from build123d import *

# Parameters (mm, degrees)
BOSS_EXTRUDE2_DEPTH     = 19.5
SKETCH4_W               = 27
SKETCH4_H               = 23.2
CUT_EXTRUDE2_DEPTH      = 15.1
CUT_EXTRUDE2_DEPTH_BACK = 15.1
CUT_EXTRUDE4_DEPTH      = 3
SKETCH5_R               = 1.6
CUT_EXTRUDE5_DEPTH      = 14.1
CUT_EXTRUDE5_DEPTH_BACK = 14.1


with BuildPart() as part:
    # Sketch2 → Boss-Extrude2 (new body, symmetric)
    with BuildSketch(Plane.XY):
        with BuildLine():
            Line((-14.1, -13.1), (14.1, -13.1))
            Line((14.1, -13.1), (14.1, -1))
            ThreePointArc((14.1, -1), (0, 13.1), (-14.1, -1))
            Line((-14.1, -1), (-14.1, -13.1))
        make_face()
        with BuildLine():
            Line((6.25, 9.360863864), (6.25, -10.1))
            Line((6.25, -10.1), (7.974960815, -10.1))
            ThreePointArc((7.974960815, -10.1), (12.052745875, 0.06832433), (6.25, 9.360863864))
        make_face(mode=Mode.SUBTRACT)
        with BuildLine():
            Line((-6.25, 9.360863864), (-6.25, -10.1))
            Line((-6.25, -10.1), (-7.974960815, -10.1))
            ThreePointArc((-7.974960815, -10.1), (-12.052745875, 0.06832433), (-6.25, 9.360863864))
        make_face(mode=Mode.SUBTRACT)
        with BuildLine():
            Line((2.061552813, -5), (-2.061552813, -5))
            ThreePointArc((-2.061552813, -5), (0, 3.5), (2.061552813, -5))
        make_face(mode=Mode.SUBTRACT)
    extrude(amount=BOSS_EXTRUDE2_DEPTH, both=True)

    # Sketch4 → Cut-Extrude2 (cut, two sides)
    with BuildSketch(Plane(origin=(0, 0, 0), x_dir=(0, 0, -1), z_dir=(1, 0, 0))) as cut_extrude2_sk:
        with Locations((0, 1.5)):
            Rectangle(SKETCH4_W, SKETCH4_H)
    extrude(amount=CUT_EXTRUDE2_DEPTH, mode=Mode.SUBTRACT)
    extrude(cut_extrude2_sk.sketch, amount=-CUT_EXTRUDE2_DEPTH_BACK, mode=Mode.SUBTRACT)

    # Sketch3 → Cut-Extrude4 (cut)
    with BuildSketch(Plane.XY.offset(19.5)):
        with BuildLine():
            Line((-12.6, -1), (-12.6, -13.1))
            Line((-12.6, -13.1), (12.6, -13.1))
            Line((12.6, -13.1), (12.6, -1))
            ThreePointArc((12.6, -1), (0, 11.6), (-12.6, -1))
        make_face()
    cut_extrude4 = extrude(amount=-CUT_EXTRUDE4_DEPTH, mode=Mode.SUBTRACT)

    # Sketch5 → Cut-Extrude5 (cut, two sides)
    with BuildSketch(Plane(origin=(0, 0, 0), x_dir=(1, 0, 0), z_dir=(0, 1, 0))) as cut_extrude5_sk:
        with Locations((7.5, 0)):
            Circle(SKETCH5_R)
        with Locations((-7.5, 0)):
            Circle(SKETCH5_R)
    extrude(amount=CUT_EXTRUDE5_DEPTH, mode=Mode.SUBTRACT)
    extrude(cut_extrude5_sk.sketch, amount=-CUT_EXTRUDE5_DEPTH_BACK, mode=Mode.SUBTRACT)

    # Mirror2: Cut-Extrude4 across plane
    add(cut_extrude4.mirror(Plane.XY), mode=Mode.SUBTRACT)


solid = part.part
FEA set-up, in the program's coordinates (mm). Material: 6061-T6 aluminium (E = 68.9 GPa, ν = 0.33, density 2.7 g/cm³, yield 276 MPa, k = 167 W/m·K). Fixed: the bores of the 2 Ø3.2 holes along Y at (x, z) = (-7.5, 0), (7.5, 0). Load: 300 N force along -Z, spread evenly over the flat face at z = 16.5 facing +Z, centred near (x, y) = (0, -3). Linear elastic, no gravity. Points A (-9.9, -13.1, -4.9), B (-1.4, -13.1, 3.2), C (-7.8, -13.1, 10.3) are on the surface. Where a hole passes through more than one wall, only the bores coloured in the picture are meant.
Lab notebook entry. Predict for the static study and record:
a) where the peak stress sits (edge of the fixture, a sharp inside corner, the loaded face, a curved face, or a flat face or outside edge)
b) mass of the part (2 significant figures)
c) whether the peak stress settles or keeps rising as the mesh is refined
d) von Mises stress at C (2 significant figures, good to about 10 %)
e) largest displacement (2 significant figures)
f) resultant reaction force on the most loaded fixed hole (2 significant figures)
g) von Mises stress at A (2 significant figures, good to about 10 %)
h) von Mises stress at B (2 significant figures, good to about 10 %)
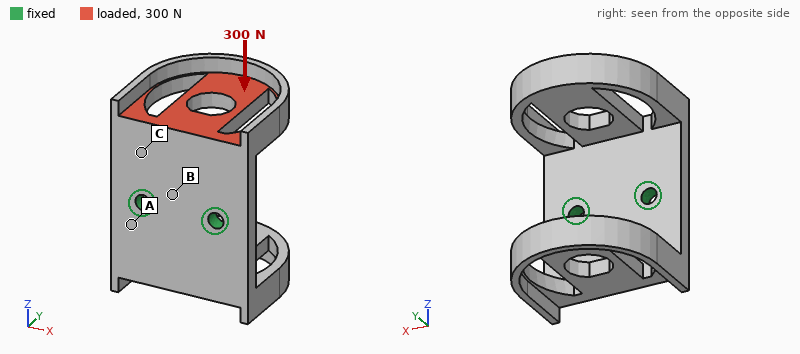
edge of the fixture
14 g
keeps rising
52 MPa
0.32 mm
150 N
7.1 MPa
44 MPa
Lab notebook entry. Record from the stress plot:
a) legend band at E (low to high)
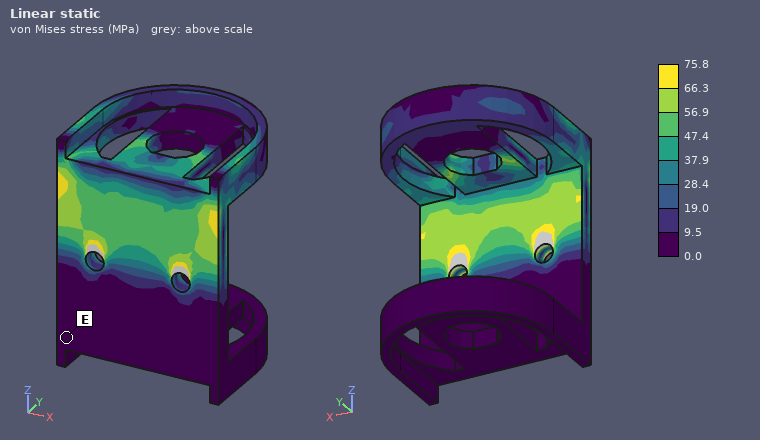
0.0 to 9.5 MPa
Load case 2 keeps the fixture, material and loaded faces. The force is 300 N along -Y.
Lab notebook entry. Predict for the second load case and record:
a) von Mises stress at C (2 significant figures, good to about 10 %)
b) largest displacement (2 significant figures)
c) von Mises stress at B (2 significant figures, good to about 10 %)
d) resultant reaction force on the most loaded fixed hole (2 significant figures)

39 MPa
0.26 mm
65 MPa
150 N
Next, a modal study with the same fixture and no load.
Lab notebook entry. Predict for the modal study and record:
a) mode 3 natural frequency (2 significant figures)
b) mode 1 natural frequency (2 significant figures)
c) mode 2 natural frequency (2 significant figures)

4000 Hz
2400 Hz
2500 Hz
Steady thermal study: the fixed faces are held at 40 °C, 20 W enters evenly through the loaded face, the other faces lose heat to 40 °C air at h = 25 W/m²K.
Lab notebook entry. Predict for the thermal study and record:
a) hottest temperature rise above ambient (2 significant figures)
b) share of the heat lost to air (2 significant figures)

45 K
7.4 %
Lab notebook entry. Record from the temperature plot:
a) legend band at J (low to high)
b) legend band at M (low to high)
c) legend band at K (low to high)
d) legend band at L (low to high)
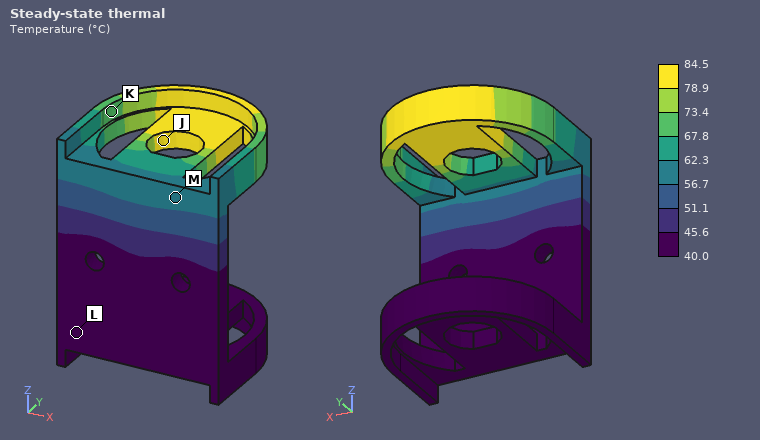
78.9 to 84.5 °C
56.7 to 62.3 °C
67.8 to 73.4 °C
40.0 to 45.6 °C
